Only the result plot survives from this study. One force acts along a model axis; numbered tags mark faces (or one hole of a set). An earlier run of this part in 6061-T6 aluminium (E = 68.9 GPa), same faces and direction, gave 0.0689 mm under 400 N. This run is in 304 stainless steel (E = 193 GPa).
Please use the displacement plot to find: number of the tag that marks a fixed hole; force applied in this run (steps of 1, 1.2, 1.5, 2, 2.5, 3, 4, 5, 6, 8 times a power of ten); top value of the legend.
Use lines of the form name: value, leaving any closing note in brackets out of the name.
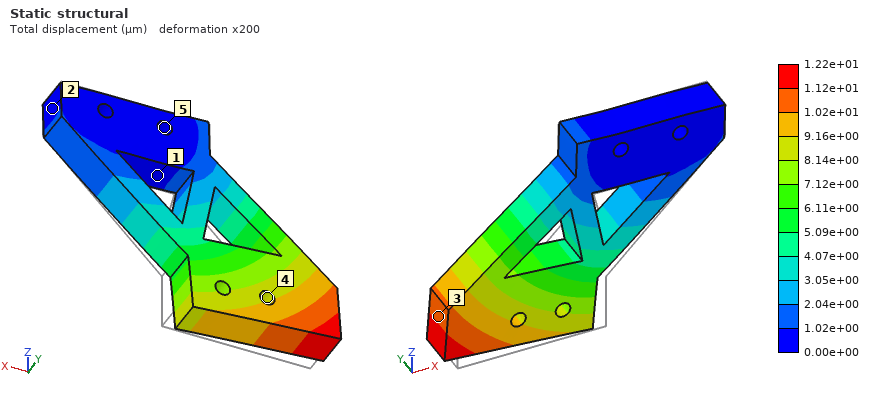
number of the tag that marks a fixed hole: 5
force applied in this run: 200 N
top value of the legend: 1.22e+01 µm
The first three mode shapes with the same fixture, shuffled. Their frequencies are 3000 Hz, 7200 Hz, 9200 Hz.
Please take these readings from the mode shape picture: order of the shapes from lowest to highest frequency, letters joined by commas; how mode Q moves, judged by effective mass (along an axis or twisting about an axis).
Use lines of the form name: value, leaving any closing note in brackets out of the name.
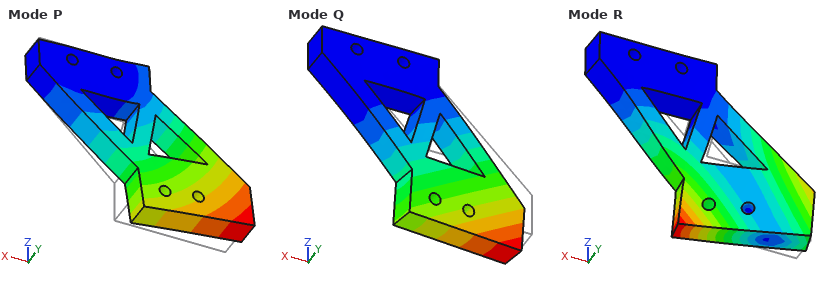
order of the shapes from lowest to highest frequency, letters joined by commas: Q, P, R
how mode Q moves, judged by effective mass: along Y
